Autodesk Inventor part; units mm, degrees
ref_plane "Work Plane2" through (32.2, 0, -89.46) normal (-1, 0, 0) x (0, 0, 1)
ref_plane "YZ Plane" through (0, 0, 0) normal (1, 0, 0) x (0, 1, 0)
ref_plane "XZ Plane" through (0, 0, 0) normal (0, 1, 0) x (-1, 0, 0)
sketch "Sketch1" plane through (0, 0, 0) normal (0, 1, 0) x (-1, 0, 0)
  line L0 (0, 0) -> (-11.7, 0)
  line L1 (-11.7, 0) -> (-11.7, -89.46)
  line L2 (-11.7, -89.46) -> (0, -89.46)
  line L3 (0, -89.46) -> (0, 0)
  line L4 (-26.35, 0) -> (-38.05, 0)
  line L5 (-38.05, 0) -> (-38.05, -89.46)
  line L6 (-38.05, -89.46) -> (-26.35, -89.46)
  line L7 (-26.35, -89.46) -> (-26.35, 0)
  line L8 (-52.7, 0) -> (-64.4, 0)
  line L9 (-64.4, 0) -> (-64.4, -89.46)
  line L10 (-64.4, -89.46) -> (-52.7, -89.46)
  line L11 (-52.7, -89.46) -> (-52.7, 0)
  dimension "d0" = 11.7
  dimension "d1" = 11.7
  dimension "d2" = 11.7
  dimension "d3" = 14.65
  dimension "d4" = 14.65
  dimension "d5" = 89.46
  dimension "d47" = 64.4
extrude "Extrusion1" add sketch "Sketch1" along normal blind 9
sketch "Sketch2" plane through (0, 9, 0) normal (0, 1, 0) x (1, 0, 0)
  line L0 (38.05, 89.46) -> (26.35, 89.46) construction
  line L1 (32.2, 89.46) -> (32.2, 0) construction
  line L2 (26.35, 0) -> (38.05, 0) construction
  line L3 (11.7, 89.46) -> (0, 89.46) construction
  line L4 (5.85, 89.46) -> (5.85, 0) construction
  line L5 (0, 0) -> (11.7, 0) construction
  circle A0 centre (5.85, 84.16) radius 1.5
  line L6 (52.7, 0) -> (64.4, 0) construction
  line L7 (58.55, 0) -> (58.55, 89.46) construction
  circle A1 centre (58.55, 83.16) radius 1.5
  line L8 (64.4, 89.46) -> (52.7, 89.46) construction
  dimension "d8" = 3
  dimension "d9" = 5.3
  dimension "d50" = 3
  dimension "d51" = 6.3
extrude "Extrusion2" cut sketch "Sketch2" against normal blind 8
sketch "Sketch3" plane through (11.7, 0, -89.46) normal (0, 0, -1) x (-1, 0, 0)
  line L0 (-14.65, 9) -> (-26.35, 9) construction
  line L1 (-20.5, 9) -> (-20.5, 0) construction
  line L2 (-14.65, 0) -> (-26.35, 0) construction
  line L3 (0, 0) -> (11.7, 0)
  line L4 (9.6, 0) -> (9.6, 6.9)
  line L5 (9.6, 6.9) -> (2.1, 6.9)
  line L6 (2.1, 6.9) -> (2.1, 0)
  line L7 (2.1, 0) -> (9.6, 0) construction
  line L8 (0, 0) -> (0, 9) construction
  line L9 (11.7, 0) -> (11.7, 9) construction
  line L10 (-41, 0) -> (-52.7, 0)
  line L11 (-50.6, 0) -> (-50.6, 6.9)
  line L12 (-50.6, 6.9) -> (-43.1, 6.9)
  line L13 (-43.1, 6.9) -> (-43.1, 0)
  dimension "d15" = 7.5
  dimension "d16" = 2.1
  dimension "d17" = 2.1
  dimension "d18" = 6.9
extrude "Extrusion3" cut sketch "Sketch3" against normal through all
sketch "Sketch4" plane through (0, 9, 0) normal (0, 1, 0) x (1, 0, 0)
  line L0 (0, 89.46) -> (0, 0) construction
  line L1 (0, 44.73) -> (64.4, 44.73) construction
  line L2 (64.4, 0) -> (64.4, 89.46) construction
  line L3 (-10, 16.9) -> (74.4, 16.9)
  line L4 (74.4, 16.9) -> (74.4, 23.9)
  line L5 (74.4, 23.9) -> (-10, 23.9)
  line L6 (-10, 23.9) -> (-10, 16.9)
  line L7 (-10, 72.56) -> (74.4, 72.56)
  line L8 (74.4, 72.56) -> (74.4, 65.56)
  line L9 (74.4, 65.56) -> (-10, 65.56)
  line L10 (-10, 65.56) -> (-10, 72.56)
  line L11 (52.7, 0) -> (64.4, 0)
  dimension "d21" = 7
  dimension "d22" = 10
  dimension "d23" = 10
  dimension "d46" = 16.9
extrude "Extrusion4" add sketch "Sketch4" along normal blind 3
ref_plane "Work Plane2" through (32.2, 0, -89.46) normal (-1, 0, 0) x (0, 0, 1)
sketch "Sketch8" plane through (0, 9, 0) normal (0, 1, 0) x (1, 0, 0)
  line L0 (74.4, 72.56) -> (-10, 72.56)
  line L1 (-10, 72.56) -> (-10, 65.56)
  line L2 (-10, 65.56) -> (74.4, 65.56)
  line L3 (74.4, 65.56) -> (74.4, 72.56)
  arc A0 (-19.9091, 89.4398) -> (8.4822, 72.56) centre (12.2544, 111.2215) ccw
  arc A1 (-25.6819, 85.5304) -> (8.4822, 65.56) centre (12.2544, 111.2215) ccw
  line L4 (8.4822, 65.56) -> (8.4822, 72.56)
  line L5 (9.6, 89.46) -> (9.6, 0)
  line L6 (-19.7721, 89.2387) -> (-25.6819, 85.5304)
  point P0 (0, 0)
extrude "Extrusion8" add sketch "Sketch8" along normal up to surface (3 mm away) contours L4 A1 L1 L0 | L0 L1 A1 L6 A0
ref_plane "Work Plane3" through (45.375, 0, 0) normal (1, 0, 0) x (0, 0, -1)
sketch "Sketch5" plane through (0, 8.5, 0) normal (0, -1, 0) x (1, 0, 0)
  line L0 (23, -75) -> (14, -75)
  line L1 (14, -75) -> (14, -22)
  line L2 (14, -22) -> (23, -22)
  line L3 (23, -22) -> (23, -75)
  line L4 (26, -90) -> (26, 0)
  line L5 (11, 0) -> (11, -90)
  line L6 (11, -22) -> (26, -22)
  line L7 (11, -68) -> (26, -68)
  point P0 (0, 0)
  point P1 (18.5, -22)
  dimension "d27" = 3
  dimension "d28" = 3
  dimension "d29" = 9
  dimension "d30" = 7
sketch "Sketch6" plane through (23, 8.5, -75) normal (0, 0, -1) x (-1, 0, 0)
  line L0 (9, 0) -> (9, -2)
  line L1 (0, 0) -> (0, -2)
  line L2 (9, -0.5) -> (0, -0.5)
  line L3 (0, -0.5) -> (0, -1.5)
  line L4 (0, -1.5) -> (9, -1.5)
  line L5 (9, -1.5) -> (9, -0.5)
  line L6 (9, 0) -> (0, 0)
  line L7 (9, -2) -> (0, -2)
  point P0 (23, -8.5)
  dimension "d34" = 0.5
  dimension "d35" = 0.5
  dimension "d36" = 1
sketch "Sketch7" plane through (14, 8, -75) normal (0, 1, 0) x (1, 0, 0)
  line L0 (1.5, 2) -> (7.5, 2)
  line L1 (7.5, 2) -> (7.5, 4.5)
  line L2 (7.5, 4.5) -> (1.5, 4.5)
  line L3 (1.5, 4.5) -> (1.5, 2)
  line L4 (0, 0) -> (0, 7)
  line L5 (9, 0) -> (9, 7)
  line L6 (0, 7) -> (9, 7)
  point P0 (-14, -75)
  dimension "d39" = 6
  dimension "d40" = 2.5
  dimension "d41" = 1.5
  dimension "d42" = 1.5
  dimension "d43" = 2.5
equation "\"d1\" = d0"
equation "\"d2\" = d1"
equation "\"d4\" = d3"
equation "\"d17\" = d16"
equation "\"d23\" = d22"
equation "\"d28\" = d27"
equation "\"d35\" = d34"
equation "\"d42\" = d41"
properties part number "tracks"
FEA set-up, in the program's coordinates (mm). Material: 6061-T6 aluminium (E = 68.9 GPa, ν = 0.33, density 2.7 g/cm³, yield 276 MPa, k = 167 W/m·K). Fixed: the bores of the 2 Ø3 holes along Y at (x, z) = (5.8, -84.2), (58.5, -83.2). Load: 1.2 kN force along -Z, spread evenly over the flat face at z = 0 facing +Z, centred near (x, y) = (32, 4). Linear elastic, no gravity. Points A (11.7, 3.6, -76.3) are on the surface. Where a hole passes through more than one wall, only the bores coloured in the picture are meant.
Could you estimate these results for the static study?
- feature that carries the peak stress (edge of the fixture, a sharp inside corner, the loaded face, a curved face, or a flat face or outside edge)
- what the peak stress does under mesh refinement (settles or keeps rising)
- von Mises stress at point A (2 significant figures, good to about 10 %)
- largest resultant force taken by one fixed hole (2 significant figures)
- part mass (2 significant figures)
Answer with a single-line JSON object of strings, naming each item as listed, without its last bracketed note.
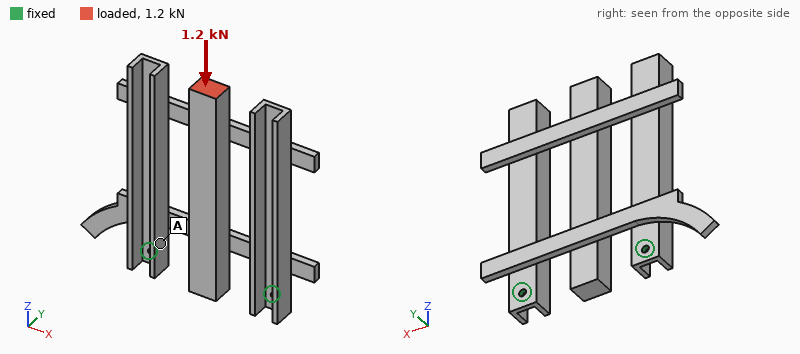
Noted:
{"feature that carries the peak stress": "edge of the fixture", "what the peak stress does under mesh refinement": "keeps rising", "von Mises stress at point A": "23 MPa", "largest resultant force taken by one fixed hole": "610 N", "part mass": "62 g"}
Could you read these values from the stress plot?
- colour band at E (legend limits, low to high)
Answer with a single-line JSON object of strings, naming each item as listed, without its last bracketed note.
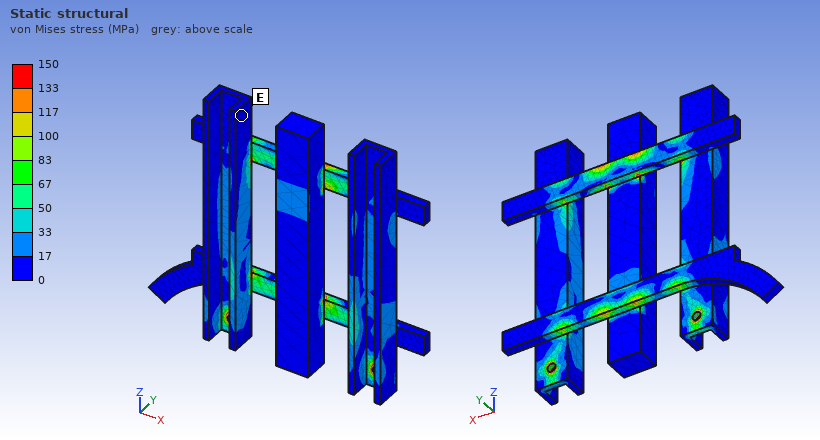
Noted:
{"colour band at E": "0 to 17 MPa"}
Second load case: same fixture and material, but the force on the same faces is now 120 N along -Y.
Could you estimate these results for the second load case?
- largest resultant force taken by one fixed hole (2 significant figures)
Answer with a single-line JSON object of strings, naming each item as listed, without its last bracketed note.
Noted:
{"largest resultant force taken by one fixed hole": "61 N"}
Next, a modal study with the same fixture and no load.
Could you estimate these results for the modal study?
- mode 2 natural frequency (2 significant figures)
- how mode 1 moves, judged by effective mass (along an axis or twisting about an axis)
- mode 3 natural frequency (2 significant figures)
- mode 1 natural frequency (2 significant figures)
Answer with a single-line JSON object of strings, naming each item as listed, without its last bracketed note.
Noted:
{"mode 2 natural frequency": "900 Hz", "how mode 1 moves, judged by effective mass": "along Y", "mode 3 natural frequency": "1500 Hz", "mode 1 natural frequency": "390 Hz"}
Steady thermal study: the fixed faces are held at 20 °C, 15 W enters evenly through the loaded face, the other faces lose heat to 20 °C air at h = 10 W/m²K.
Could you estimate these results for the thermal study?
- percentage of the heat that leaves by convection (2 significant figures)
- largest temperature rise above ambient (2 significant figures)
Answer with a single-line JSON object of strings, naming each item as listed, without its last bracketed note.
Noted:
{"percentage of the heat that leaves by convection": "26 %", "largest temperature rise above ambient": "63 K"}
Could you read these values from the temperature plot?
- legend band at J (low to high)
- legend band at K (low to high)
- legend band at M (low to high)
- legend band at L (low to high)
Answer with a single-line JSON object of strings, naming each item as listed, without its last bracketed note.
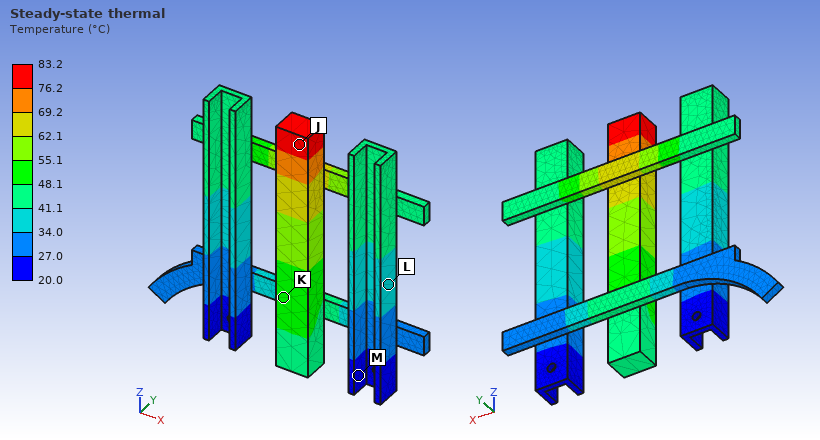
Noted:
{"legend band at J": "76.2 to 83.2 °C", "legend band at K": "48.1 to 55.1 °C", "legend band at M": "20.0 to 27.0 °C", "legend band at L": "34.0 to 41.1 °C"}
